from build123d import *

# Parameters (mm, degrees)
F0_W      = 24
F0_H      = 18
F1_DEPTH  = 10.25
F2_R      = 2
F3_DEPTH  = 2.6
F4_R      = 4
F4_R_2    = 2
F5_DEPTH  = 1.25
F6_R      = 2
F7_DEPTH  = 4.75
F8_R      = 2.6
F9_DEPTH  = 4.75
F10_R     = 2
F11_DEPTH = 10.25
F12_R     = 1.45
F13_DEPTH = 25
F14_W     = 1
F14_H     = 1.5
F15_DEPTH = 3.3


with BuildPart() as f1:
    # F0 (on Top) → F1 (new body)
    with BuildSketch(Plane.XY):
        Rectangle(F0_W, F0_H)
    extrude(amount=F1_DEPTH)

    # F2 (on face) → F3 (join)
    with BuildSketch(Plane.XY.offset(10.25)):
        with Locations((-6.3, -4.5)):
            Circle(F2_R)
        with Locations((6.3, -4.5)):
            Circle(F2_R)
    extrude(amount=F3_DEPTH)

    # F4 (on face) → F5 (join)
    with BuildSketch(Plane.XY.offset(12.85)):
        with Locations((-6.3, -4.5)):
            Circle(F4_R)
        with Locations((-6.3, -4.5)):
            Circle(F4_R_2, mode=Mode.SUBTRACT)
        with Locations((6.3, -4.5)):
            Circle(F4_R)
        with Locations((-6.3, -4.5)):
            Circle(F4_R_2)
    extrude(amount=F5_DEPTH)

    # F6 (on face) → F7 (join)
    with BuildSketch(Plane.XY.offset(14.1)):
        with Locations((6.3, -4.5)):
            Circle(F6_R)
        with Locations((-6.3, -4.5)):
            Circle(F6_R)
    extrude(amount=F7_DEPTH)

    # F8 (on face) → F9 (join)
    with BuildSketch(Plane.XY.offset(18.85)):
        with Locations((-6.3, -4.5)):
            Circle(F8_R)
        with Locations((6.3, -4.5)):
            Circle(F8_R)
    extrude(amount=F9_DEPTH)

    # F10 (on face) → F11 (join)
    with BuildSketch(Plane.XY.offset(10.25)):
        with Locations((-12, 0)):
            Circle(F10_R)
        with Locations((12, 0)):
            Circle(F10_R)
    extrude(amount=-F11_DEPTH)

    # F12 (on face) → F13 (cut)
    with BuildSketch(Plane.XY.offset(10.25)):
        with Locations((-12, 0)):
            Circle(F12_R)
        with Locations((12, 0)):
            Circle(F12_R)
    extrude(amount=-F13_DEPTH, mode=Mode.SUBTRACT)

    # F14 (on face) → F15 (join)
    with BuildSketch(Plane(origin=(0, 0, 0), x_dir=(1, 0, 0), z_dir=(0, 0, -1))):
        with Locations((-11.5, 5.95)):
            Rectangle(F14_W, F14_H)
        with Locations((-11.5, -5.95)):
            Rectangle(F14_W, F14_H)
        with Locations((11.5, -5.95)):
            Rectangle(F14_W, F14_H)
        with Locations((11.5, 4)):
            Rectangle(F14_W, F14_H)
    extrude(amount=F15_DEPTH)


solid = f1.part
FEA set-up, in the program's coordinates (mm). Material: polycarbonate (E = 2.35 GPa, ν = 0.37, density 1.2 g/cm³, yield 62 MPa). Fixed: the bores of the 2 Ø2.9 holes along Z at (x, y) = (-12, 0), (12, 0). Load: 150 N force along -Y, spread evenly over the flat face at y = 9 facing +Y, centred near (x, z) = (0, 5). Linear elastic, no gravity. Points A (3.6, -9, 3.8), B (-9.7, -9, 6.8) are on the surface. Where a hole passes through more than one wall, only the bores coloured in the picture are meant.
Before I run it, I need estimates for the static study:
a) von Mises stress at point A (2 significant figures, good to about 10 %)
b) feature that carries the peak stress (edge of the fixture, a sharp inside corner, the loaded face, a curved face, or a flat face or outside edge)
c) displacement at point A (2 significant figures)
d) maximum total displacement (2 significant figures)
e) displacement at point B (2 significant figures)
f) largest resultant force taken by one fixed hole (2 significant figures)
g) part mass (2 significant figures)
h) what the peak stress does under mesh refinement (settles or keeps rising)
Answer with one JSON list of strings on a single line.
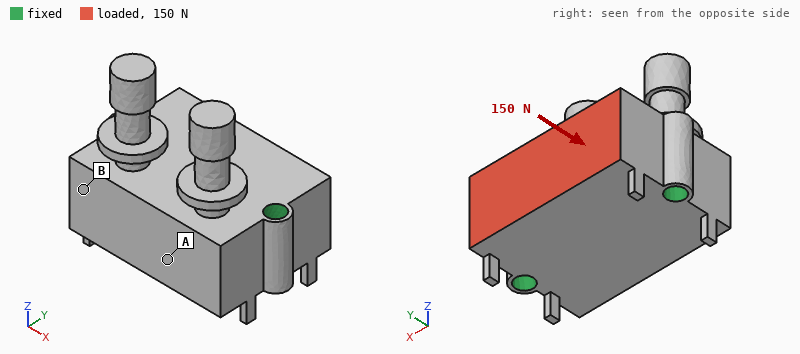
["0.62 MPa", "edge of the fixture", "3.7 µm", "6.4 µm", "2.6 µm", "76 N", "5.9 g", "keeps rising"]
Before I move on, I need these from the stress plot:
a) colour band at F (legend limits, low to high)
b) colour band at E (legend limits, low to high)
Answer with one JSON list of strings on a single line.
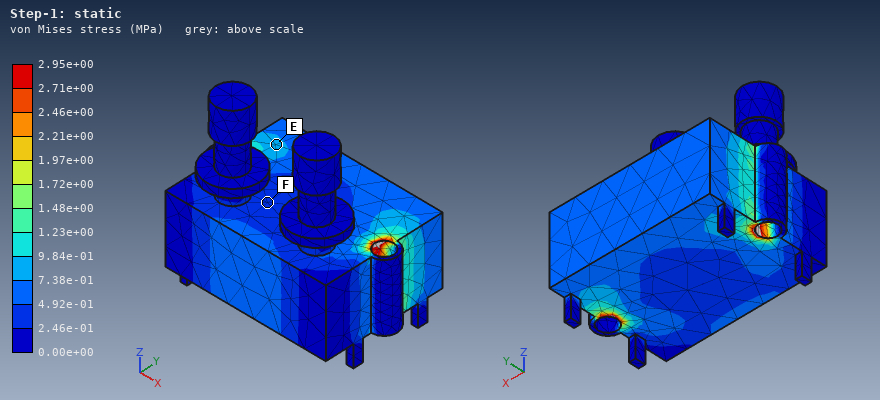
["2.46e-01 to 4.92e-01 MPa", "7.38e-01 to 9.84e-01 MPa"]
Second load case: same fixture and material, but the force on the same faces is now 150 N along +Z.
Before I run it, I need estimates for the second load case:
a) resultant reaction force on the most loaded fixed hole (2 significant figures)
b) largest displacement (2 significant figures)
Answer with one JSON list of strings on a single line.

["75 N", "36 µm"]
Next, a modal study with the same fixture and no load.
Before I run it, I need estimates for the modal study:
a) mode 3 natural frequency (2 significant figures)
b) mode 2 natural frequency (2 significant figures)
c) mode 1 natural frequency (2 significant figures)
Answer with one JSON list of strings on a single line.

["3000 Hz", "3000 Hz", "3000 Hz"]
